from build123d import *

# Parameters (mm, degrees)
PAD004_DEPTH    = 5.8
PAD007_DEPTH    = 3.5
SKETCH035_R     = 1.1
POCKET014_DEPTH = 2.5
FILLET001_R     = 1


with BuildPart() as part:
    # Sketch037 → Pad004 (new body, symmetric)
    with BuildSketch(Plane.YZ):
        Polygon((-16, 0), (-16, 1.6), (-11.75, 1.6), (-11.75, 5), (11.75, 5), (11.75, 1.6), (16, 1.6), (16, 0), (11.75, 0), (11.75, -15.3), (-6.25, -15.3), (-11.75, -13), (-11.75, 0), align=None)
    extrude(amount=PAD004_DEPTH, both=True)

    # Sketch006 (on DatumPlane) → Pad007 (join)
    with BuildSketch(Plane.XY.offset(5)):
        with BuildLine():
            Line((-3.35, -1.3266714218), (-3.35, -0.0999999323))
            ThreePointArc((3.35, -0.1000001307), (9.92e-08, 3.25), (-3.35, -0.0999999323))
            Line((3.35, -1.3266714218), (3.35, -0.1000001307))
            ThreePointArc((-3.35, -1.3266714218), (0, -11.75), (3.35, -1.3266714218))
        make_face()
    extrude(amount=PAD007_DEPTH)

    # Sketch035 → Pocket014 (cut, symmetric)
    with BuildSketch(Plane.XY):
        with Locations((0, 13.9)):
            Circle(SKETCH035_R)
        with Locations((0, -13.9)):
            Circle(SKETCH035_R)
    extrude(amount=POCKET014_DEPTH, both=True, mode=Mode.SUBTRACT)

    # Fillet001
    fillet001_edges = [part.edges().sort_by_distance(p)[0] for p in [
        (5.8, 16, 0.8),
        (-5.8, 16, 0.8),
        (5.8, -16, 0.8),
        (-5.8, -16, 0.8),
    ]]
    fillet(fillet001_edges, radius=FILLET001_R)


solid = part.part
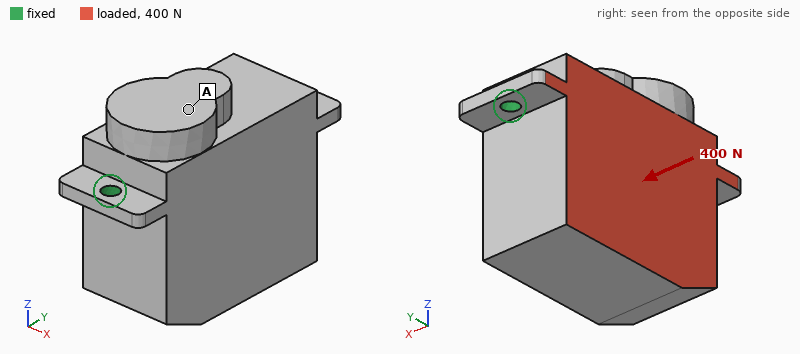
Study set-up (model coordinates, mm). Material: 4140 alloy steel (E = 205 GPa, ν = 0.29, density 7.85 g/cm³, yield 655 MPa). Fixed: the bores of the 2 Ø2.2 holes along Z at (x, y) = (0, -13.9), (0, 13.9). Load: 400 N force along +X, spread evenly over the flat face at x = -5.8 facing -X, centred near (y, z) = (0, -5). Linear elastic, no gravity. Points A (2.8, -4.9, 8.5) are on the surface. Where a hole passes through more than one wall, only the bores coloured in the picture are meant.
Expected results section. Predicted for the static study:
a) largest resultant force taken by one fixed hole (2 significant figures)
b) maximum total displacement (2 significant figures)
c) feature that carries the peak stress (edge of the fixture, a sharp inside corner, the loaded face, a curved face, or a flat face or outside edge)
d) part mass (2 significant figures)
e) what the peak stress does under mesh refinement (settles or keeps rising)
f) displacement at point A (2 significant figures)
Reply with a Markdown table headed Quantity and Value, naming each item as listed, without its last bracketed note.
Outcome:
| Quantity | Value |
|---|---|
| largest resultant force taken by one fixed hole | 200 N |
| maximum total displacement | 31 µm |
| feature that carries the peak stress | edge of the fixture |
| part mass | 47 g |
| what the peak stress does under mesh refinement | keeps rising |
| displacement at point A | 13 µm |
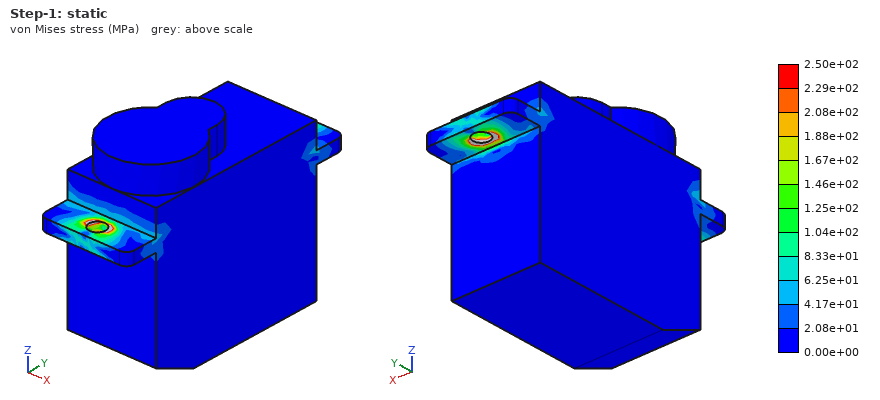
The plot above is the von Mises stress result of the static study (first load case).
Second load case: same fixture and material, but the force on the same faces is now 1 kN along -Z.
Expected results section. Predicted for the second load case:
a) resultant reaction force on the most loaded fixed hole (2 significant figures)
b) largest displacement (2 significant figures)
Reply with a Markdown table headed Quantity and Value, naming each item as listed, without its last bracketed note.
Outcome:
| Quantity | Value |
|---|---|
| resultant reaction force on the most loaded fixed hole | 510 N |
| largest displacement | 77 µm |
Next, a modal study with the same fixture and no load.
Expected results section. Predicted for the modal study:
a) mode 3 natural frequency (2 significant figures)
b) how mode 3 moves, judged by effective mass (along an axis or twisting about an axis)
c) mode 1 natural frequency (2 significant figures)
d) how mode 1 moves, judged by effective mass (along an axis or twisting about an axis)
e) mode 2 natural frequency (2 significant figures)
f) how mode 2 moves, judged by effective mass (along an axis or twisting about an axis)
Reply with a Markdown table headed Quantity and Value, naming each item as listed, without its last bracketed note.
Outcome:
| Quantity | Value |
|---|---|
| mode 3 natural frequency | 16 kHz |
| how mode 3 moves, judged by effective mass | along Y |
| mode 1 natural frequency | 3000 Hz |
| how mode 1 moves, judged by effective mass | along X |
| mode 2 natural frequency | 14 kHz |
| how mode 2 moves, judged by effective mass | along Z |
